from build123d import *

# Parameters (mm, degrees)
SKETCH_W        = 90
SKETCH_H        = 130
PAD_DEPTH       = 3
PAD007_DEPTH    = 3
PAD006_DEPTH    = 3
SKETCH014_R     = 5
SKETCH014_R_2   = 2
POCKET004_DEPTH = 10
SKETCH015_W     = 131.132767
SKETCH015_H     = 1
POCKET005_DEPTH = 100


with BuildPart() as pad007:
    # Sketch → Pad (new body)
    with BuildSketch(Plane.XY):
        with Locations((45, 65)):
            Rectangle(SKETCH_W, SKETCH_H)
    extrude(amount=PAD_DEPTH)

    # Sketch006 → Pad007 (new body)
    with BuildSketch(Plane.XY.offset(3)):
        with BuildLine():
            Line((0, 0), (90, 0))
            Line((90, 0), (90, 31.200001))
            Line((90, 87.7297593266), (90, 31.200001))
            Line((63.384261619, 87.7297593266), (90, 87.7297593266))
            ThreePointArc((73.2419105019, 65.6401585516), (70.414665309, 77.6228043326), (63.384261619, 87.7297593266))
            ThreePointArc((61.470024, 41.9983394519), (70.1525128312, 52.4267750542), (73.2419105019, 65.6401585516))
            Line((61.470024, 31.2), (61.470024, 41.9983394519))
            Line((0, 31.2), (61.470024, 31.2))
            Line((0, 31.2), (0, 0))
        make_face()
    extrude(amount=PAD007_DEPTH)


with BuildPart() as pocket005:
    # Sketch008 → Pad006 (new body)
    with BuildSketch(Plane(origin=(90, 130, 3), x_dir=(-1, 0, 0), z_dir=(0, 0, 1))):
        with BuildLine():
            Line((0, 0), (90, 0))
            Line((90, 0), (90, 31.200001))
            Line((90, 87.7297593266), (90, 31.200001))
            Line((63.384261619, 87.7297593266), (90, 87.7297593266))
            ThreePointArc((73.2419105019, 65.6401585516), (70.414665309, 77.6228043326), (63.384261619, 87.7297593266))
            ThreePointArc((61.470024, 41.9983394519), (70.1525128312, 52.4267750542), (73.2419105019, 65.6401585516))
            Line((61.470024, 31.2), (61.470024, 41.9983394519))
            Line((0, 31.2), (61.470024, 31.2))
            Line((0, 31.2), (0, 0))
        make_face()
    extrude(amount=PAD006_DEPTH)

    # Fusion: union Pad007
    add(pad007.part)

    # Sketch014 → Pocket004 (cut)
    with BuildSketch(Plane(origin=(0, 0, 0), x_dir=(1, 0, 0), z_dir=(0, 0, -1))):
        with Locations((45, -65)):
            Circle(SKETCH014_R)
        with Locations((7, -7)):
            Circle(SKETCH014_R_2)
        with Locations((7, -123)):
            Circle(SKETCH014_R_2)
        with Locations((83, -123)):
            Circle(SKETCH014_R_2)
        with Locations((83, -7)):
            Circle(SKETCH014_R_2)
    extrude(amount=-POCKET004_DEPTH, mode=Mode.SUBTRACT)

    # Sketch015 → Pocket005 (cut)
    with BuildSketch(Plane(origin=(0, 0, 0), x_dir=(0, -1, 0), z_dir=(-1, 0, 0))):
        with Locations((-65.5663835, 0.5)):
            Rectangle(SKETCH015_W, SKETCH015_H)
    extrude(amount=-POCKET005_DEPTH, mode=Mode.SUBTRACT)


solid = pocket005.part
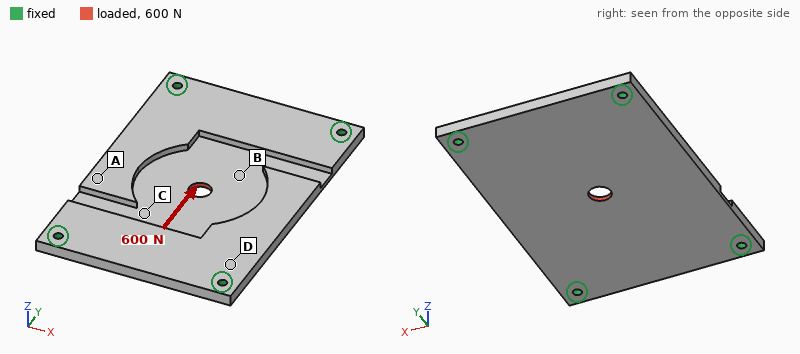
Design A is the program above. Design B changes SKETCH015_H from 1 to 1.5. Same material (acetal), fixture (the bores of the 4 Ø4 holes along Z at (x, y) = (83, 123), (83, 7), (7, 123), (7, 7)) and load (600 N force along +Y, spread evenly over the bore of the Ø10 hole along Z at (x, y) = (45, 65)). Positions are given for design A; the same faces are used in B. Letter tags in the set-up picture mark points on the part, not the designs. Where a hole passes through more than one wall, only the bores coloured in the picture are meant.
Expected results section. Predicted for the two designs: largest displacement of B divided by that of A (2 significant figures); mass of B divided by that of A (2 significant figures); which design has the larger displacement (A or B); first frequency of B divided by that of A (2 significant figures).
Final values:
1.1
0.94
B
0.96
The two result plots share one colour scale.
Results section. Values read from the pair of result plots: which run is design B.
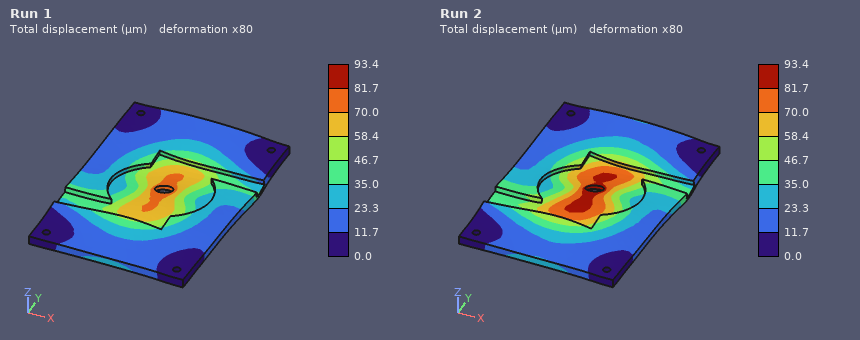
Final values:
Run 2
